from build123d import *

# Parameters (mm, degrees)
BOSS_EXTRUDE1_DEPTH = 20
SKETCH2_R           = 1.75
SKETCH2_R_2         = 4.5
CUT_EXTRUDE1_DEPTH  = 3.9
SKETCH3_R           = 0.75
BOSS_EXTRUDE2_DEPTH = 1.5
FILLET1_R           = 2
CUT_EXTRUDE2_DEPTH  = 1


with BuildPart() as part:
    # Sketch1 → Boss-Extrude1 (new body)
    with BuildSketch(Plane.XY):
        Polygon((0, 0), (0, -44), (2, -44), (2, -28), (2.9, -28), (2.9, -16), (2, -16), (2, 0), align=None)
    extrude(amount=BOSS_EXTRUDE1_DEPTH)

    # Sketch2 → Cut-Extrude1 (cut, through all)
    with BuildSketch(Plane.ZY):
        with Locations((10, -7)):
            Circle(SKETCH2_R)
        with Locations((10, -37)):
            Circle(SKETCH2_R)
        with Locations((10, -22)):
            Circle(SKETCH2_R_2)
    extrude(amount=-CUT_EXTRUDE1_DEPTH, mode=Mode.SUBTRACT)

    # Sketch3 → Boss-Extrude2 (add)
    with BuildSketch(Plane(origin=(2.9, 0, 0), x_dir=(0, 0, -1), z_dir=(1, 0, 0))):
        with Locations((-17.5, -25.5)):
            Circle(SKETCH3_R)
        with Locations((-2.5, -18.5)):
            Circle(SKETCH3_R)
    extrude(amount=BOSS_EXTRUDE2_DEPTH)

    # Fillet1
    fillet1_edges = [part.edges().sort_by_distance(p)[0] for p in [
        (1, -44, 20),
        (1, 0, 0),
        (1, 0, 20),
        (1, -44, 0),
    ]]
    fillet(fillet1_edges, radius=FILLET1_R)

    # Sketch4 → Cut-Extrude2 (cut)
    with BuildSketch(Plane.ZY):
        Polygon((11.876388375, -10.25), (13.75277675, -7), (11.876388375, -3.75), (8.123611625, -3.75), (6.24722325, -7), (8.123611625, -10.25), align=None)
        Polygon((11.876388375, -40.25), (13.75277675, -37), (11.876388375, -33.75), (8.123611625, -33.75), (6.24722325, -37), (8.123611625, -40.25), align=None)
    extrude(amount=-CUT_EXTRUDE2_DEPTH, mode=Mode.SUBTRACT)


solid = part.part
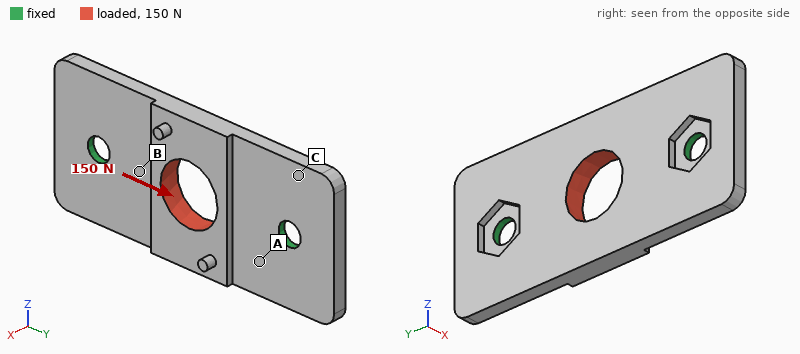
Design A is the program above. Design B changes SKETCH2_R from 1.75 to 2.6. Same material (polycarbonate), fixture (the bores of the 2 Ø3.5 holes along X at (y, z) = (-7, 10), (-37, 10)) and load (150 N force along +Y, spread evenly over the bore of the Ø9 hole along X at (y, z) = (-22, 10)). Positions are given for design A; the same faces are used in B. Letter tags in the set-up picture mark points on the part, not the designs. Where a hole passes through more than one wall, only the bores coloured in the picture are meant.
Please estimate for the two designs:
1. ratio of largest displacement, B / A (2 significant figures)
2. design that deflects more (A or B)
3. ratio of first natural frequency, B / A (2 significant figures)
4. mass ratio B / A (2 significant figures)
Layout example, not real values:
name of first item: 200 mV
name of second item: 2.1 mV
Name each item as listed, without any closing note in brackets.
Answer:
ratio of largest displacement, B / A: 0.78
design that deflects more: A
ratio of first natural frequency, B / A: 1.3
mass ratio B / A: 0.99
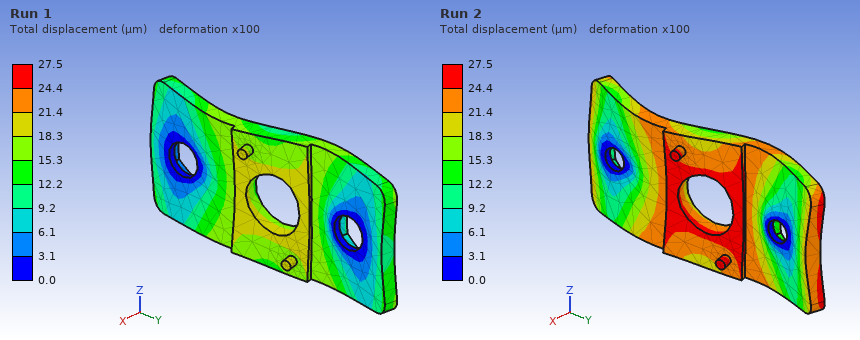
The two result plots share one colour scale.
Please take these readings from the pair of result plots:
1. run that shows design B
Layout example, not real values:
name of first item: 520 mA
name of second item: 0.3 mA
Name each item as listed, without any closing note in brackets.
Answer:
run that shows design B: Run 1
